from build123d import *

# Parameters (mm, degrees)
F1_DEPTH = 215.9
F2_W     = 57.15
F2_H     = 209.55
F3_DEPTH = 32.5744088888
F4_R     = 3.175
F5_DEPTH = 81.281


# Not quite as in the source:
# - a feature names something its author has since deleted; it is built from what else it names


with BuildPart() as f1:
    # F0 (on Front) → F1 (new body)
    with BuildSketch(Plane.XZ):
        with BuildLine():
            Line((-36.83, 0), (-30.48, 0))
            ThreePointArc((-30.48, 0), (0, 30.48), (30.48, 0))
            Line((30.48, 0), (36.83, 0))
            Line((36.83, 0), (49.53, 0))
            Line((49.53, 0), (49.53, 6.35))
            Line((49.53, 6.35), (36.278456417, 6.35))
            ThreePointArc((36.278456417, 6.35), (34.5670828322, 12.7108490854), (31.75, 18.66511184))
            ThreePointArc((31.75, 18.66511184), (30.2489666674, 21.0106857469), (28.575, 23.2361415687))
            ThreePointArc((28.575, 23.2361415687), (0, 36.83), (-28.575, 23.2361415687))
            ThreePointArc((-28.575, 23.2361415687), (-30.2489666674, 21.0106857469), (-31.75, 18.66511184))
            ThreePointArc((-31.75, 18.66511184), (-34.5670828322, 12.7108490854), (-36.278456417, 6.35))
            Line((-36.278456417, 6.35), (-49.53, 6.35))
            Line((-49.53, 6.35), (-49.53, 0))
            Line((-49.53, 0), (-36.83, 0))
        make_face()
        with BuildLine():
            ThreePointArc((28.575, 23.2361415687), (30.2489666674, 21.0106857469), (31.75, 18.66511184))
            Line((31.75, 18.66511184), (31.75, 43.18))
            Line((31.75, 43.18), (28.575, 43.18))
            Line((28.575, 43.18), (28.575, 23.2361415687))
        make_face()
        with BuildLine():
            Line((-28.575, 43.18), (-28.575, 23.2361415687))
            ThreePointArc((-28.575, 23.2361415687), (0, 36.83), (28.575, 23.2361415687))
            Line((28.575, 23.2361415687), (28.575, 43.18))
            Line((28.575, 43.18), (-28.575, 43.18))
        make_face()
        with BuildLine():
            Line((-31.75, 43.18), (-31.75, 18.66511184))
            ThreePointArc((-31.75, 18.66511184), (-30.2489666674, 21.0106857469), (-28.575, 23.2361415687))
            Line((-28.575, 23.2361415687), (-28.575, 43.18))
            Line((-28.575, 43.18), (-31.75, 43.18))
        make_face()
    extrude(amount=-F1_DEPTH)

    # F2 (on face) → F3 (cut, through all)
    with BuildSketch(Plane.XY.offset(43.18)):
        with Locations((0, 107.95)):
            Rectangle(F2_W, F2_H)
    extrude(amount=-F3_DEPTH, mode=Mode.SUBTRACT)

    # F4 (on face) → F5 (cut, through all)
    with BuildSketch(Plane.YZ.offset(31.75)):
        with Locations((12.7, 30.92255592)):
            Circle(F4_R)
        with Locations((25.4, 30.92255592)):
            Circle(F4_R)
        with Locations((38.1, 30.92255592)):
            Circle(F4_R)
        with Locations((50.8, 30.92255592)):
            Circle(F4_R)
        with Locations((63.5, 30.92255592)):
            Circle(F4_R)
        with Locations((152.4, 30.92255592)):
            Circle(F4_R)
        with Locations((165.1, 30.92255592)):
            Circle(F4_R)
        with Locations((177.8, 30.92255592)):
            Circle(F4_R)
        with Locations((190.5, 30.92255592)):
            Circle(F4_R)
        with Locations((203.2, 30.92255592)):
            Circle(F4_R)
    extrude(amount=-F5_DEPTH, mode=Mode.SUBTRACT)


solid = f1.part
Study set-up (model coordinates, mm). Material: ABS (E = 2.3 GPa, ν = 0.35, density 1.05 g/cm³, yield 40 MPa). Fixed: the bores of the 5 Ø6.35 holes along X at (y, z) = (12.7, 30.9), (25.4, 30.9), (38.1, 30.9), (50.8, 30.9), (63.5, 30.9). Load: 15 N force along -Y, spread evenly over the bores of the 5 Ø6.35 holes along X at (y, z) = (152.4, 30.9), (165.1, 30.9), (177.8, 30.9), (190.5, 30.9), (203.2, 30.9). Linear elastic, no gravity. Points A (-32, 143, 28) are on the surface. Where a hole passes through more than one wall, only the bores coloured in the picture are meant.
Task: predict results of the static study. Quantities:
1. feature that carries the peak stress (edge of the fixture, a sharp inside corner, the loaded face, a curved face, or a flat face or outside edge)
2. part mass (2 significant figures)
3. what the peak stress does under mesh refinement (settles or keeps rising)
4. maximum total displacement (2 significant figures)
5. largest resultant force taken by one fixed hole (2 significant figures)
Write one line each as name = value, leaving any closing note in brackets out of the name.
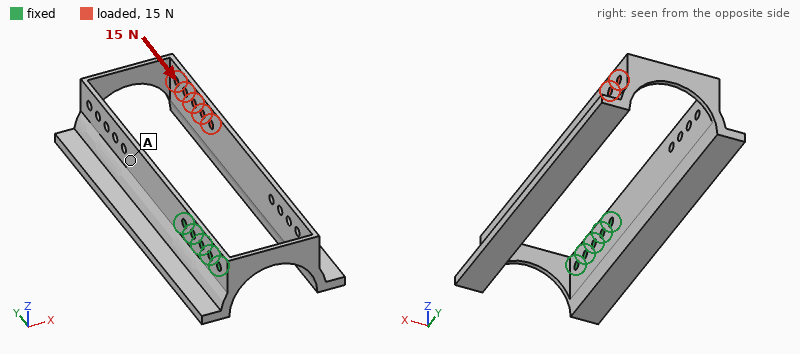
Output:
feature that carries the peak stress = edge of the fixture
part mass = 130 g
what the peak stress does under mesh refinement = keeps rising
maximum total displacement = 2.3 mm
largest resultant force taken by one fixed hole = 14 N
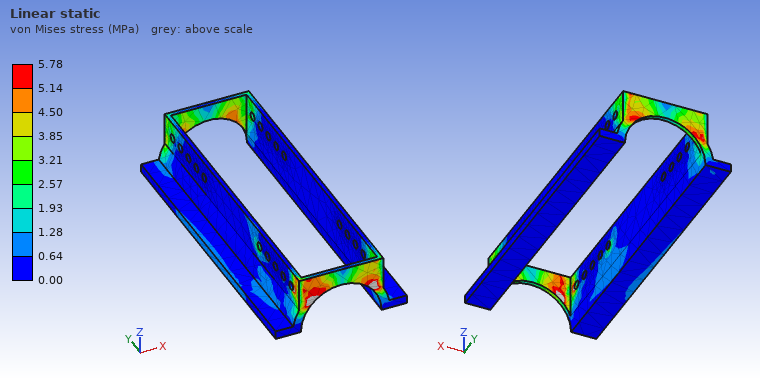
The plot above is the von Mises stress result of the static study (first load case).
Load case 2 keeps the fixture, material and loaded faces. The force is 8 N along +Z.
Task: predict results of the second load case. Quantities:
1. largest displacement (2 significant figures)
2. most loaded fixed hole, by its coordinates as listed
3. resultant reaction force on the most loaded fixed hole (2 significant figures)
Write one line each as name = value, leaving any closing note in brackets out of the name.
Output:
largest displacement = 2.6 mm
most loaded fixed hole, by its coordinates as listed = (63.5, 30.9)
resultant reaction force on the most loaded fixed hole = 31 N
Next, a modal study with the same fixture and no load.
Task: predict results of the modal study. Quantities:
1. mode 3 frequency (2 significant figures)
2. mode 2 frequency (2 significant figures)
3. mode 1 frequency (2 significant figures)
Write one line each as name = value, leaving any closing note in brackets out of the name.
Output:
mode 3 frequency = 69 Hz
mode 2 frequency = 54 Hz
mode 1 frequency = 45 Hz
